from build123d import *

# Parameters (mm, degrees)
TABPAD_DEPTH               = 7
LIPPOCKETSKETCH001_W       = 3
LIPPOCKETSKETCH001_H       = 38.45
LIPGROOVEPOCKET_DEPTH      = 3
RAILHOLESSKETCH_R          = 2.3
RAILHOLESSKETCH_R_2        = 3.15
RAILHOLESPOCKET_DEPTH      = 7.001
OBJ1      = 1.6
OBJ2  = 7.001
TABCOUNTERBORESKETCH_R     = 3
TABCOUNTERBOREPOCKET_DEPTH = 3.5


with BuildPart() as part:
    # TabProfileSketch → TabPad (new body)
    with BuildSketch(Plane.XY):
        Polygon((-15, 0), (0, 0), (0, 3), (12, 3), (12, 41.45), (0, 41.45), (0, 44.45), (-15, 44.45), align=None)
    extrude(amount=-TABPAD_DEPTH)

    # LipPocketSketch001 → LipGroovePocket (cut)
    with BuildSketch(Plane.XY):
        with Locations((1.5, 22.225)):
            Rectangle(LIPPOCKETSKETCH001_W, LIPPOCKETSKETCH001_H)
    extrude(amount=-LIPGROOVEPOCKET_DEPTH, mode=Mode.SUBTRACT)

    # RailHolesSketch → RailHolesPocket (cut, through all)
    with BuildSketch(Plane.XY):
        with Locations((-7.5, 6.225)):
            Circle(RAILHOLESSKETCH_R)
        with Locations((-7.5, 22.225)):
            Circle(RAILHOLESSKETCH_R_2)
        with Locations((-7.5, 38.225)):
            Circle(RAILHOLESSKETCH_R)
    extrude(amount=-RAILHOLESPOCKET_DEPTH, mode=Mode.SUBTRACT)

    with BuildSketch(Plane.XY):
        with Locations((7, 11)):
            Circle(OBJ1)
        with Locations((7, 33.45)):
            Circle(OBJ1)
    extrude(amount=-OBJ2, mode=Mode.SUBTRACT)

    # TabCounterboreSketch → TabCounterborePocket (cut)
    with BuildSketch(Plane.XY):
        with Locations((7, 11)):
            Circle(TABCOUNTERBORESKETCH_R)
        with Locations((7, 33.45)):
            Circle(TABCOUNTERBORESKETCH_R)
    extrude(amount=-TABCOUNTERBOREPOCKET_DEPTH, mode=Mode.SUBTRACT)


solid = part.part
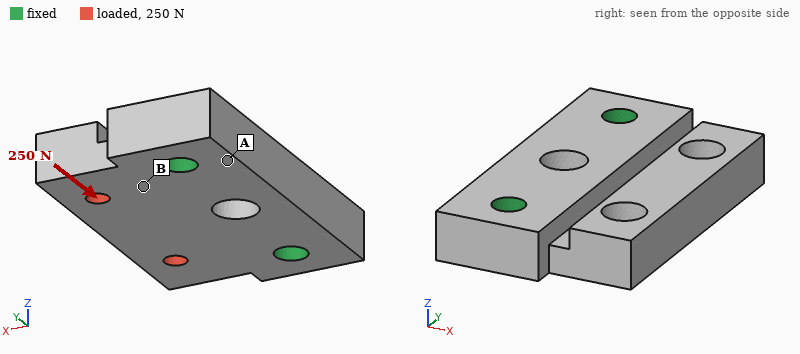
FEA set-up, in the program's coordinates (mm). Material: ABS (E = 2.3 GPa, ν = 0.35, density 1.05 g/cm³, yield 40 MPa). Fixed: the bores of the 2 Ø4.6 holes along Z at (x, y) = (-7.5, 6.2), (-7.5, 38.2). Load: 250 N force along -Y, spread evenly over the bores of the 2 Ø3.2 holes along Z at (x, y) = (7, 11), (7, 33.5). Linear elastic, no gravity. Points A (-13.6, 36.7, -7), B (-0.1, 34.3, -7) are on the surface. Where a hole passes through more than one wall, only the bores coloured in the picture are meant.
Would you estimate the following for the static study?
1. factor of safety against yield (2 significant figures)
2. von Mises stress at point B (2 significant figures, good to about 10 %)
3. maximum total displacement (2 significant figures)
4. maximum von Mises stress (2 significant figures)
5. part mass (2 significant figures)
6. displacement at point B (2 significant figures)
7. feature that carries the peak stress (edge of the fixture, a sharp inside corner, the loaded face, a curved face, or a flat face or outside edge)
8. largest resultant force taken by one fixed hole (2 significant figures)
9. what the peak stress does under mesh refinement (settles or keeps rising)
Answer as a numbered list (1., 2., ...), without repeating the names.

1. 5.2
2. 2.9 MPa
3. 40 µm
4. 7.7 MPa
5. 7.2 g
6. 12 µm
7. the loaded face
8. 160 N
9. settles
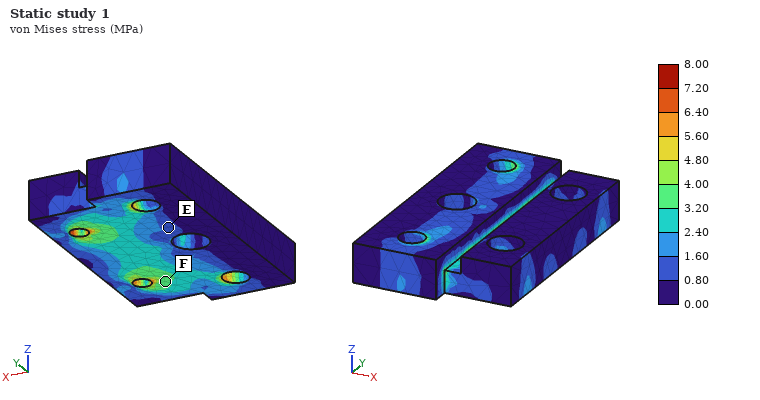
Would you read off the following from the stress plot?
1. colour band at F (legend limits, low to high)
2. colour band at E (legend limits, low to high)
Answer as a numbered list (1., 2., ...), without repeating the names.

1. 3.20 to 4.00 MPa
2. 0.80 to 1.60 MPa
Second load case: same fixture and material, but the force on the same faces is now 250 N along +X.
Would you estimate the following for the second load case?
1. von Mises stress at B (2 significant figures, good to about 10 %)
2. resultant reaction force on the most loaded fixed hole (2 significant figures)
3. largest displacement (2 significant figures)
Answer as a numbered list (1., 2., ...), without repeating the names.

1. 3.2 MPa
2. 130 N
3. 43 µm
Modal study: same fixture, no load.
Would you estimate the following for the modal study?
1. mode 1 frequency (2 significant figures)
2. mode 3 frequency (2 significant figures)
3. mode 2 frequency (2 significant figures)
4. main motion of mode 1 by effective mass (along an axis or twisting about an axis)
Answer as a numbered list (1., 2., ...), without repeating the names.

1. 2900 Hz
2. 7900 Hz
3. 5000 Hz
4. along Z
